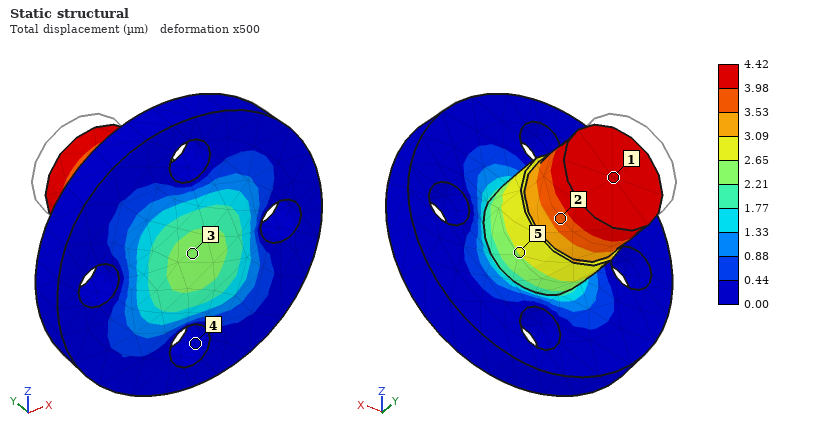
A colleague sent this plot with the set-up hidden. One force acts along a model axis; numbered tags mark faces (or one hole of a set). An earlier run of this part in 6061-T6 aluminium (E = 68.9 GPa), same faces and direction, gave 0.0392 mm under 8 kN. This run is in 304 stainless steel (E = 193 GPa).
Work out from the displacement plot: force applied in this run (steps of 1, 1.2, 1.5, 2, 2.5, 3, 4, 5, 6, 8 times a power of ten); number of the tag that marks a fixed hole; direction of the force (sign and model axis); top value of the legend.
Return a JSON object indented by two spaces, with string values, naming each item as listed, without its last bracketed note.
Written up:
{
  "force applied in this run": "2.5 kN",
  "number of the tag that marks a fixed hole": "4",
  "direction of the force": "-Y",
  "top value of the legend": "4.42 µm"
}
